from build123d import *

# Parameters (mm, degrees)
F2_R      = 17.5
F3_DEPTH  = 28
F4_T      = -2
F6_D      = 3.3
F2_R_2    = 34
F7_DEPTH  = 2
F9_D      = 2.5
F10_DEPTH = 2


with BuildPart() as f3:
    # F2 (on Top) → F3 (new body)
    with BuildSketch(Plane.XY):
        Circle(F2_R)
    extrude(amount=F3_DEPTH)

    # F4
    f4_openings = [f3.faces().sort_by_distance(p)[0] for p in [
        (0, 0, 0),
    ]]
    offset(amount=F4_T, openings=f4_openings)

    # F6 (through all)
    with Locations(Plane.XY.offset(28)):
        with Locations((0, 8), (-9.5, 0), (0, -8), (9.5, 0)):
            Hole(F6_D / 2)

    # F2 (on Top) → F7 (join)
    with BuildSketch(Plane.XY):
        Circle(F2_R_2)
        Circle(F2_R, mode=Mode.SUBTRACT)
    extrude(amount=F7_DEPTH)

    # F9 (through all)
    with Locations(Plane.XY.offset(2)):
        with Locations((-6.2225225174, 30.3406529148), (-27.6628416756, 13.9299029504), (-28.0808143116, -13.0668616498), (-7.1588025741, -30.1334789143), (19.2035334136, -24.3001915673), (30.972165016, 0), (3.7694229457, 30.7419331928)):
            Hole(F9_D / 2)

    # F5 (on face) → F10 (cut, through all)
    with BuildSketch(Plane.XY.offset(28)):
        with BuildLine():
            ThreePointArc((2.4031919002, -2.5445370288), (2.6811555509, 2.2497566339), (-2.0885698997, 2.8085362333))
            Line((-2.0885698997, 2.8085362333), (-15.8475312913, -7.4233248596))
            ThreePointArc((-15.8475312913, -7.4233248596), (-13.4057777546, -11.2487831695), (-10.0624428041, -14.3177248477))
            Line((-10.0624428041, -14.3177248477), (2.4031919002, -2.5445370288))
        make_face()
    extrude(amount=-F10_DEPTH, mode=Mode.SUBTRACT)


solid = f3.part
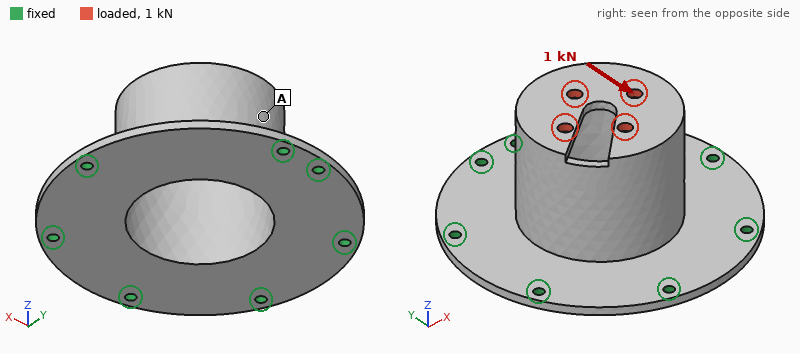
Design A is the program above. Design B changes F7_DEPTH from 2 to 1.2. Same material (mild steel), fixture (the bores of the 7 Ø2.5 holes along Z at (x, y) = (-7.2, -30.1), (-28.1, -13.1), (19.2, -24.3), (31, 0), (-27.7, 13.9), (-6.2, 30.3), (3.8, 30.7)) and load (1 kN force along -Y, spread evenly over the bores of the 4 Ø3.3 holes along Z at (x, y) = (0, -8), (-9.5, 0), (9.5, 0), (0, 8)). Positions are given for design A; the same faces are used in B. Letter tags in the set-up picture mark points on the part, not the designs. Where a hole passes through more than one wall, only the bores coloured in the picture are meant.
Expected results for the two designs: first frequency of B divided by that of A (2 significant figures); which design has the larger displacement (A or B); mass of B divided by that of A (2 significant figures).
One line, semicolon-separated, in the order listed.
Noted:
0.56; B; 0.83
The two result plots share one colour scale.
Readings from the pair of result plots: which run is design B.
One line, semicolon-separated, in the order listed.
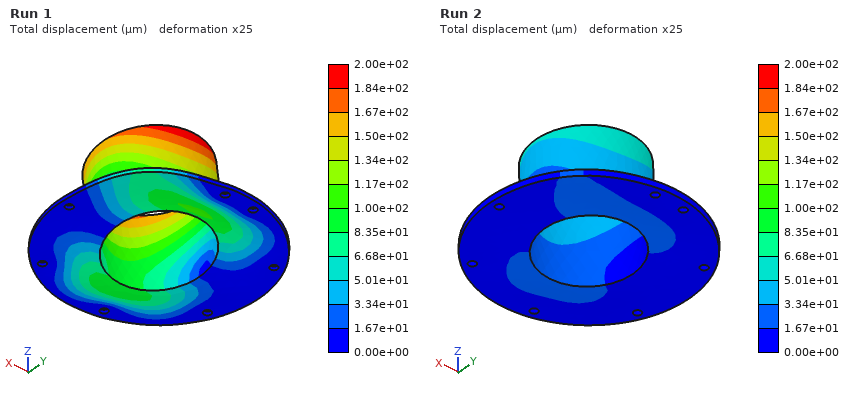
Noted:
Run 1
